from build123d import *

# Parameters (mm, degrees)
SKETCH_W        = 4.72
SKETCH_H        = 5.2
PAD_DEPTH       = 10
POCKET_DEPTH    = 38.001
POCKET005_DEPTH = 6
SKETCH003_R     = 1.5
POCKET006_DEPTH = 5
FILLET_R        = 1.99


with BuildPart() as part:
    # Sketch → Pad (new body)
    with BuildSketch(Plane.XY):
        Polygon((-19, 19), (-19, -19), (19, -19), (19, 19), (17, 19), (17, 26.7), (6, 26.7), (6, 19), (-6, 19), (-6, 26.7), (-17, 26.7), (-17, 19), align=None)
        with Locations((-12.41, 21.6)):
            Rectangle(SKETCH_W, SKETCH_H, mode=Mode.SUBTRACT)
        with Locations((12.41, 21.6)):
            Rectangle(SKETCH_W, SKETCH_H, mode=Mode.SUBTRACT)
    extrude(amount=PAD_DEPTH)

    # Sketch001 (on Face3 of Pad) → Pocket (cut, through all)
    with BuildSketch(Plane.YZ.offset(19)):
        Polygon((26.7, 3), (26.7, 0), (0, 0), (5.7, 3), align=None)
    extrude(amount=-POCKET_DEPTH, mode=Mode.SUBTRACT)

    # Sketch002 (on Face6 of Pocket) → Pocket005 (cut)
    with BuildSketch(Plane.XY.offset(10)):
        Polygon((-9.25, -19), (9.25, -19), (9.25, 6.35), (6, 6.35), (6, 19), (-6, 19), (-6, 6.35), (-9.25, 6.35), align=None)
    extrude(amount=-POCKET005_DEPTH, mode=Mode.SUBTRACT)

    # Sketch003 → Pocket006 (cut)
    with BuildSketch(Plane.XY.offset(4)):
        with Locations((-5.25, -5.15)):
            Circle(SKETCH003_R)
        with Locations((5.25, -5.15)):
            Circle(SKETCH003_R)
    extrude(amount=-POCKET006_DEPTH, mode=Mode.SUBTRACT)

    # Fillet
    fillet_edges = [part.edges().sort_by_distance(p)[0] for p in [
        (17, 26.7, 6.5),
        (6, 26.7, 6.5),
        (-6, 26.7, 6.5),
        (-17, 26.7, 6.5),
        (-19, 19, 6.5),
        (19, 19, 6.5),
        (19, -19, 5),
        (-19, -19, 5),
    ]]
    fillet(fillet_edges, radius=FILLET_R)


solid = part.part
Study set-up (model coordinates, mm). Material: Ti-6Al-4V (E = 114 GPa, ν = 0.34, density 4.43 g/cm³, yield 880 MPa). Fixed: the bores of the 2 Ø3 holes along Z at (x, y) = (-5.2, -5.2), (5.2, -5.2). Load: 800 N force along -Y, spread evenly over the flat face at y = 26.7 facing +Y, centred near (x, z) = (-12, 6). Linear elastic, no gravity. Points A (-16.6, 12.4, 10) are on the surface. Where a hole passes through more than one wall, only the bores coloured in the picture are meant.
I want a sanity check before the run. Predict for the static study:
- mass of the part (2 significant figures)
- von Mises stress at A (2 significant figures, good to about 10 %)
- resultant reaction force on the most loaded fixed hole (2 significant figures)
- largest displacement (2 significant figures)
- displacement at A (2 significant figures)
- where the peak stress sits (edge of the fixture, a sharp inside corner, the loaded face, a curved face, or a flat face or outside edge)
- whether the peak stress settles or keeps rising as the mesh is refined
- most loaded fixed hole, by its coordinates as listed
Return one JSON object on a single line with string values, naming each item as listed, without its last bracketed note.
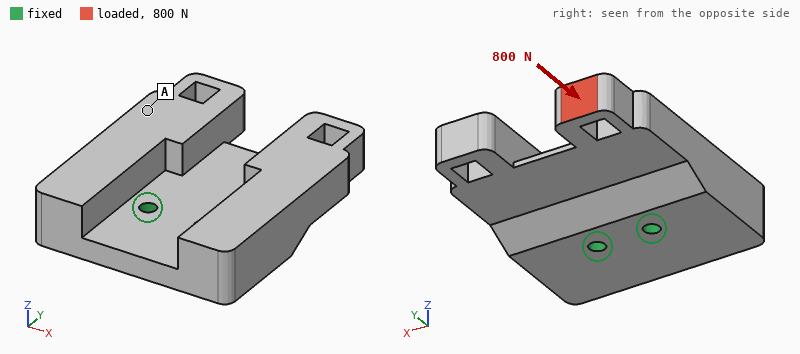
{"mass of the part": "43 g", "von Mises stress at A": "11 MPa", "resultant reaction force on the most loaded fixed hole": "1.1 kN", "largest displacement": "40 µm", "displacement at A": "23 µm", "where the peak stress sits": "edge of the fixture", "whether the peak stress settles or keeps rising as the mesh is refined": "keeps rising", "most loaded fixed hole, by its coordinates as listed": "(-5.2, -5.2)"}
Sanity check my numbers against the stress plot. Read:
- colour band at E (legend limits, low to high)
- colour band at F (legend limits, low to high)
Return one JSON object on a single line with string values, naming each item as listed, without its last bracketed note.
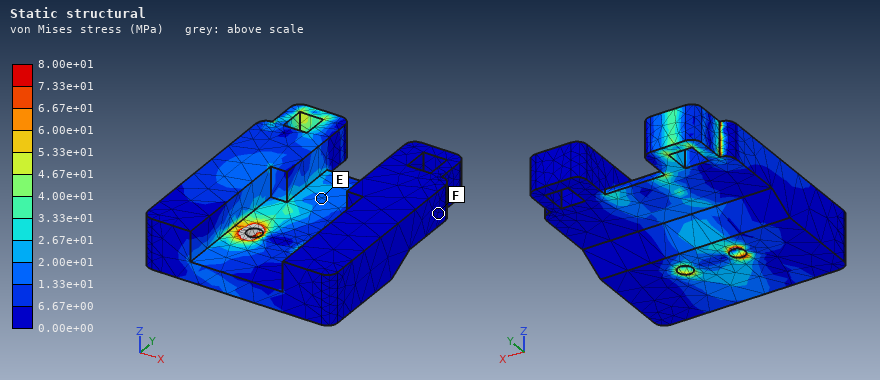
{"colour band at E": "1.33e+01 to 2.00e+01 MPa", "colour band at F": "0.00e+00 to 6.67e+00 MPa"}
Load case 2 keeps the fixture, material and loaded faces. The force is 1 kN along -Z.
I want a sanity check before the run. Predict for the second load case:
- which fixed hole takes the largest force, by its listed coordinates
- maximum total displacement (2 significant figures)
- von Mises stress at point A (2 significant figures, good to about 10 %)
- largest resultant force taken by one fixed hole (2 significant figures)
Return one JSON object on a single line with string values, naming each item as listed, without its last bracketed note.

{"which fixed hole takes the largest force, by its listed coordinates": "(-5.2, -5.2)", "maximum total displacement": "0.48 mm", "von Mises stress at point A": "140 MPa", "largest resultant force taken by one fixed hole": "1.2 kN"}
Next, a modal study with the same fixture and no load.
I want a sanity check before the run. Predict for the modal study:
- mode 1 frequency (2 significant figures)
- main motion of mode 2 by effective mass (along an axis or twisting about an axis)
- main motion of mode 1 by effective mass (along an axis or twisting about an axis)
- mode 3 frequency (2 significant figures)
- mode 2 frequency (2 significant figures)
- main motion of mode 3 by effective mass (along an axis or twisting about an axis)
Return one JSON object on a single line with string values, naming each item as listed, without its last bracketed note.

{"mode 1 frequency": "3900 Hz", "main motion of mode 2 by effective mass": "twisting about Y", "main motion of mode 1 by effective mass": "along Z", "mode 3 frequency": "6900 Hz", "mode 2 frequency": "4500 Hz", "main motion of mode 3 by effective mass": "along X"}
